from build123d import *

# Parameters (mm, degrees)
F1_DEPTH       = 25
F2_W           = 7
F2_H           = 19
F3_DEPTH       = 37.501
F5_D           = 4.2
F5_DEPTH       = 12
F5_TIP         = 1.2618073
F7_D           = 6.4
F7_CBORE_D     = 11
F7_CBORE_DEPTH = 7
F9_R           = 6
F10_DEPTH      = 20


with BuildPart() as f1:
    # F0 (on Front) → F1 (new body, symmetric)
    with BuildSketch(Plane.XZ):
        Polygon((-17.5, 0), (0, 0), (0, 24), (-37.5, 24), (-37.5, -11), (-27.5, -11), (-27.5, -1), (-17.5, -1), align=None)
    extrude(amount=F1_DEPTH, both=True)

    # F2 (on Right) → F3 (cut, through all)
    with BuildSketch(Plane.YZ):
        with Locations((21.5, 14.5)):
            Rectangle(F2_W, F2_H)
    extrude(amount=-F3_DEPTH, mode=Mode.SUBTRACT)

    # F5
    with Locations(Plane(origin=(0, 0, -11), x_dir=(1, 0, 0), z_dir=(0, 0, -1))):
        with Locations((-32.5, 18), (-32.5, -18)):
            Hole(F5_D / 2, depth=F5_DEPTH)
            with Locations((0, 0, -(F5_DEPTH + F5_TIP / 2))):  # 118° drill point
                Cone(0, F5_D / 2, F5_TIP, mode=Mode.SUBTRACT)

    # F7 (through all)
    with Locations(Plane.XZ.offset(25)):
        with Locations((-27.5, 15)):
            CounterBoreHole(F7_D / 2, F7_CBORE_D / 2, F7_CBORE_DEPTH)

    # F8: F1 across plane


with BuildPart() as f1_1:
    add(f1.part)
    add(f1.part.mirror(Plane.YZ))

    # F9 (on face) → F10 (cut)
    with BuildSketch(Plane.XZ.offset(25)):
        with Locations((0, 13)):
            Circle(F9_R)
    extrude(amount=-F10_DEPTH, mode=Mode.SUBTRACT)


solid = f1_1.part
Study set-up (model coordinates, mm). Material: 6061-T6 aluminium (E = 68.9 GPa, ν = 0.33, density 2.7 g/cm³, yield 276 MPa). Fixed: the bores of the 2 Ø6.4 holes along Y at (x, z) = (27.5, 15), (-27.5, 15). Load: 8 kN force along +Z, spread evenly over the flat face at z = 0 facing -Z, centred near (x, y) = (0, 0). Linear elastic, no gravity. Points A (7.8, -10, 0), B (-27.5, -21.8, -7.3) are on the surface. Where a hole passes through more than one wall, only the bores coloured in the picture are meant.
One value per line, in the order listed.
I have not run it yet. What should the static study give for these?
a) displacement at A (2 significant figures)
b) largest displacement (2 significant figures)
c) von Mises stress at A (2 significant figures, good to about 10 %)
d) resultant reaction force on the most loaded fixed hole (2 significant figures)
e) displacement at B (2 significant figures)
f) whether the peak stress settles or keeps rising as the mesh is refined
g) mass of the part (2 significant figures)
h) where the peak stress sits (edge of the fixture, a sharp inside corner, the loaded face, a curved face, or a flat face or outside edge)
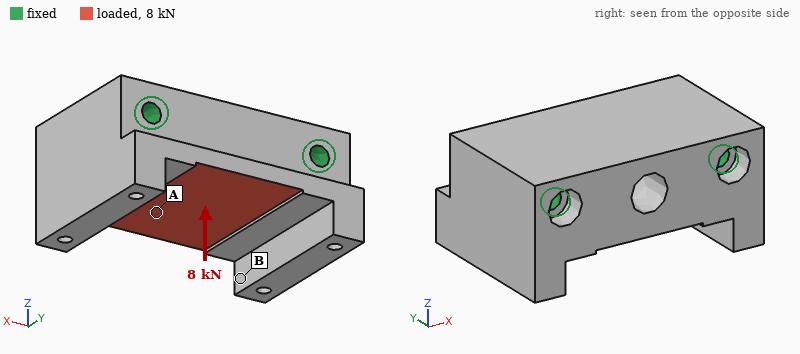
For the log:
5.8 µm
17 µm
10 MPa
4.4 kN
3.7 µm
keeps rising
230 g
edge of the fixture
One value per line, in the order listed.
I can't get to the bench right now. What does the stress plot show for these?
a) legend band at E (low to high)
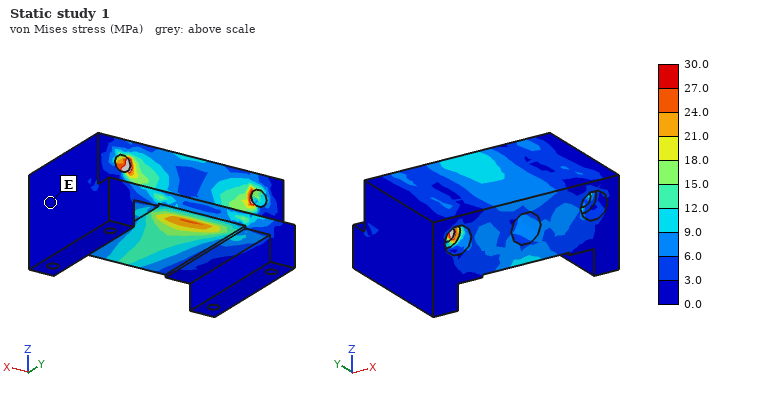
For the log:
0.0 to 3.0 MPa
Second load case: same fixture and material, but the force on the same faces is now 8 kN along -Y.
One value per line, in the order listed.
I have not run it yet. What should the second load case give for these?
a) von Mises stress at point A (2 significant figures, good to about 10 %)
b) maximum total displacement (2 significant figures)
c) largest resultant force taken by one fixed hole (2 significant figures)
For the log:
12 MPa
18 µm
4.0 kN
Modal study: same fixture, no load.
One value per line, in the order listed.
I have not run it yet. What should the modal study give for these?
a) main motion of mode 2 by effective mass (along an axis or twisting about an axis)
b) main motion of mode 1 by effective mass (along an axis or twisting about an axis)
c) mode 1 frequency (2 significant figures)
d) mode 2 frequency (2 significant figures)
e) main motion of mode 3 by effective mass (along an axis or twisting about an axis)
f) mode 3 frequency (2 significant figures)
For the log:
along Y
along Z
16 kHz
19 kHz
along X
20 kHz
